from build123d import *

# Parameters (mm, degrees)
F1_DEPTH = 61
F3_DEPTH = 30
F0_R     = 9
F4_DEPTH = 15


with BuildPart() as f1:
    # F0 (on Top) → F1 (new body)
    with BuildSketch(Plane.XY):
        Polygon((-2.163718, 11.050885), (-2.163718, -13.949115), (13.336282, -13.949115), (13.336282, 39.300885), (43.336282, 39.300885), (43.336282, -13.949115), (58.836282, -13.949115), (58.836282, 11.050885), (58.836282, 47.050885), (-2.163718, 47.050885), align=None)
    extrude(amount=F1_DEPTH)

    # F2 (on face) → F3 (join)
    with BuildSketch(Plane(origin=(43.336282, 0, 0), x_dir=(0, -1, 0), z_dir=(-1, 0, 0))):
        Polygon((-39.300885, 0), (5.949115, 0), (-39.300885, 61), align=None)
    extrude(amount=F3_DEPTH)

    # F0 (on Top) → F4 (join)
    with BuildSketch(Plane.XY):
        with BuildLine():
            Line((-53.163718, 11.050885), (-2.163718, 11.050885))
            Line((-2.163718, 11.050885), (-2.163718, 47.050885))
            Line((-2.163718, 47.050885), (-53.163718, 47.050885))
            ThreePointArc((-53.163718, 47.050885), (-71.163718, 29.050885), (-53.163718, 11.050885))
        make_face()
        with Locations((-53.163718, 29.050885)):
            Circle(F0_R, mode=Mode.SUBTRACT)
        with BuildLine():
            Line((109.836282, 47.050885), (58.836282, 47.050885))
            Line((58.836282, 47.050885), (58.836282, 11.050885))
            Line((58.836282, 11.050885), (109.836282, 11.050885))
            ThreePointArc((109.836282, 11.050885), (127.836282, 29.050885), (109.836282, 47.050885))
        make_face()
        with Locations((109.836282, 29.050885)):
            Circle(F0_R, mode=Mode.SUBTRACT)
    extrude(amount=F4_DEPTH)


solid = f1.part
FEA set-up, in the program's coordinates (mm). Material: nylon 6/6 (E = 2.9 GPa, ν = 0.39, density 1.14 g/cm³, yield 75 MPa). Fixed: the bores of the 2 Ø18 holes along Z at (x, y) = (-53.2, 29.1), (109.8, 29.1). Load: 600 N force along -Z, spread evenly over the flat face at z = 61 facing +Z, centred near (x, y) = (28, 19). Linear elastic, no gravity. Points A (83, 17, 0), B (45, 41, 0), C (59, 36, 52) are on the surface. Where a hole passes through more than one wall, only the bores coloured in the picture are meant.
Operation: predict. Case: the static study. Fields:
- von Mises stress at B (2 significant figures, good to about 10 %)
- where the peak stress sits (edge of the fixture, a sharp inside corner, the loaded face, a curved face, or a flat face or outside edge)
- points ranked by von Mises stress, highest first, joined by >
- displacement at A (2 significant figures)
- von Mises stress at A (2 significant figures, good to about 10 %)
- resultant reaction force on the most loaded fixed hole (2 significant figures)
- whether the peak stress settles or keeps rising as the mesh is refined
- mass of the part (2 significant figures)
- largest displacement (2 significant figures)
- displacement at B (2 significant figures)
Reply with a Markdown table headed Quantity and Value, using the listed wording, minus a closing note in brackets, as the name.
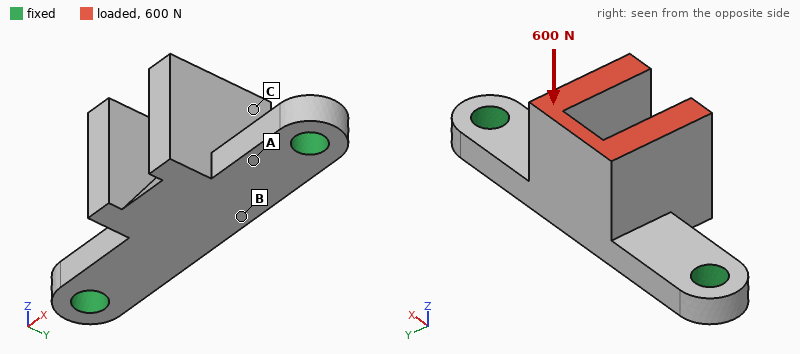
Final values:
| Quantity | Value |
|---|---|
| von Mises stress at B | 1.3 MPa |
| where the peak stress sits | edge of the fixture |
| points ranked by von Mises stress, highest first, joined by > | A > B > C |
| displacement at A | 0.084 mm |
| von Mises stress at A | 2.5 MPa |
| resultant reaction force on the most loaded fixed hole | 330 N |
| whether the peak stress settles or keeps rising as the mesh is refined | keeps rising |
| mass of the part | 270 g |
| largest displacement | 0.39 mm |
| displacement at B | 0.11 mm |
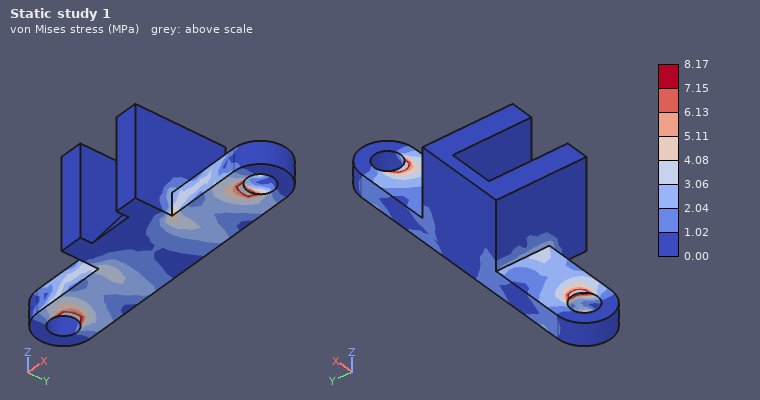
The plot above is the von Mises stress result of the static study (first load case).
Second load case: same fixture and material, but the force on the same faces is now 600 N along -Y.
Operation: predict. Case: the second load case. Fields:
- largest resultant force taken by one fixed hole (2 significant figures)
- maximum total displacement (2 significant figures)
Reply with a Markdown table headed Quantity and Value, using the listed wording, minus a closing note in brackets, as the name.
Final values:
| Quantity | Value |
|---|---|
| largest resultant force taken by one fixed hole | 310 N |
| maximum total displacement | 1.6 mm |
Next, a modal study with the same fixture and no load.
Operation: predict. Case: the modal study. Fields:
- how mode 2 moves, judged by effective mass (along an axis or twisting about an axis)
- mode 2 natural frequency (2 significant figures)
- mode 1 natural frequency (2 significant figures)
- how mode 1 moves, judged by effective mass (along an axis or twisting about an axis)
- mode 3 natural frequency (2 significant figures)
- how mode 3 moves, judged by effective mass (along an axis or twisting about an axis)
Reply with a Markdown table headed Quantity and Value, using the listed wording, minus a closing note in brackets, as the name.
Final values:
| Quantity | Value |
|---|---|
| how mode 2 moves, judged by effective mass | along Z |
| mode 2 natural frequency | 720 Hz |
| mode 1 natural frequency | 390 Hz |
| how mode 1 moves, judged by effective mass | along Y |
| mode 3 natural frequency | 1100 Hz |
| how mode 3 moves, judged by effective mass | along X |
